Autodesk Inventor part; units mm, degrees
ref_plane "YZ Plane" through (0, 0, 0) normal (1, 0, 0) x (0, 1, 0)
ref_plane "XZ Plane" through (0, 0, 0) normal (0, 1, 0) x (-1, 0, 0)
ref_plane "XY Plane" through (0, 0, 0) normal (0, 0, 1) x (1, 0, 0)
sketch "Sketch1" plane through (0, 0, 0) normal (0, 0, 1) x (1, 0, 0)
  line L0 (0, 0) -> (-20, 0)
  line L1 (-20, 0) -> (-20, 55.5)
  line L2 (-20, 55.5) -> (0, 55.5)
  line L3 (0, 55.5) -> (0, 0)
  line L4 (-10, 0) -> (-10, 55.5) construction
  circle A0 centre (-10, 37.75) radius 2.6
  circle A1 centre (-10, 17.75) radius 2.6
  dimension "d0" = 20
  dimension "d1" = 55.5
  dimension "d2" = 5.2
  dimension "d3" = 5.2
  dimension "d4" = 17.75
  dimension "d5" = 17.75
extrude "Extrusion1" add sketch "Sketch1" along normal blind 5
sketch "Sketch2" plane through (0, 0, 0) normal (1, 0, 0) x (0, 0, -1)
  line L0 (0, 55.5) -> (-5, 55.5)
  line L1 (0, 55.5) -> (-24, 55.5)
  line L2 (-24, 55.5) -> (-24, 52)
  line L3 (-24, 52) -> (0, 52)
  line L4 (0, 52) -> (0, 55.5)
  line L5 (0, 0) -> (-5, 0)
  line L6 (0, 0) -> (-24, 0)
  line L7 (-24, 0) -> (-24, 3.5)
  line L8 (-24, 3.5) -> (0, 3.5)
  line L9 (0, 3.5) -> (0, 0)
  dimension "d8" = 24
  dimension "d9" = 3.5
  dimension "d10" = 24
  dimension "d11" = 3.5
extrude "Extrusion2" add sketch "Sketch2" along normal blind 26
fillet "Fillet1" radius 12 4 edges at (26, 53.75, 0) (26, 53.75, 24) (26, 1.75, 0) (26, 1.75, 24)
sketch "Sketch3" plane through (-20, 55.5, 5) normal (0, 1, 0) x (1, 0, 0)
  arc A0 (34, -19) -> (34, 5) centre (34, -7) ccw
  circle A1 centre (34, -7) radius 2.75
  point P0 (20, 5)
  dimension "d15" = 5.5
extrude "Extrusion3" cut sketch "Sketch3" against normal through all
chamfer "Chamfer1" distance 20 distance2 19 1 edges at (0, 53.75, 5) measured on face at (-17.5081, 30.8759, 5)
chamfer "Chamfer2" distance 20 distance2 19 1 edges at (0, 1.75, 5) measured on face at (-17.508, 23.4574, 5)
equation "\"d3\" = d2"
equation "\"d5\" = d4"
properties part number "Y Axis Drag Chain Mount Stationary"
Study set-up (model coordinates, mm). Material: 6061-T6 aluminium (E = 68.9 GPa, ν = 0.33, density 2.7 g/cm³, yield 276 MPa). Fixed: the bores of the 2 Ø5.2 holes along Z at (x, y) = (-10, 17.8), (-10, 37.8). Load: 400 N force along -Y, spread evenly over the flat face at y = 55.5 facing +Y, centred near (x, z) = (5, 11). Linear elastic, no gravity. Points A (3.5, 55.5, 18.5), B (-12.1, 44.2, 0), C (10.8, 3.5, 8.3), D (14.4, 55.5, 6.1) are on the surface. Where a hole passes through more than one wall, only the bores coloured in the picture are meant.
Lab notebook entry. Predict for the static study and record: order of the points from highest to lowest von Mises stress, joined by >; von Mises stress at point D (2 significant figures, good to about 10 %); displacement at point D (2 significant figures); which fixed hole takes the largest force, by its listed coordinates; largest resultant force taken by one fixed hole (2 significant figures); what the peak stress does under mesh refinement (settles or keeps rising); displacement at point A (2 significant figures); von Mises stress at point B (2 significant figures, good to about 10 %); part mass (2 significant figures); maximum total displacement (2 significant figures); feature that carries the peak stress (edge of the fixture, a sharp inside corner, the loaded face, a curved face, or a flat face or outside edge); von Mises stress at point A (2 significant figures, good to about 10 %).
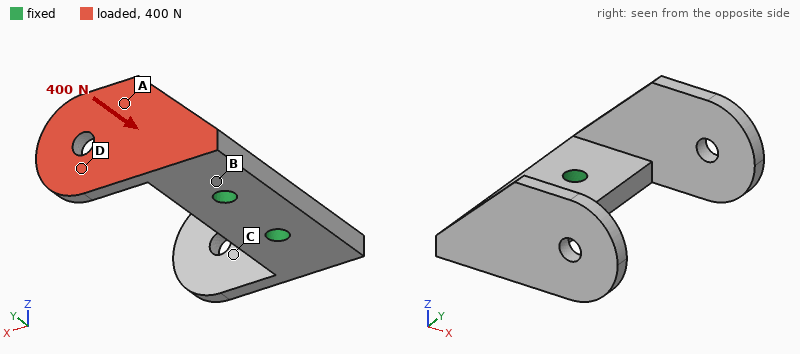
B > A > D > C
17 MPa
0.15 mm
(-10, 37.8)
390 N
keeps rising
0.16 mm
39 MPa
28 g
0.35 mm
a sharp inside corner
28 MPa
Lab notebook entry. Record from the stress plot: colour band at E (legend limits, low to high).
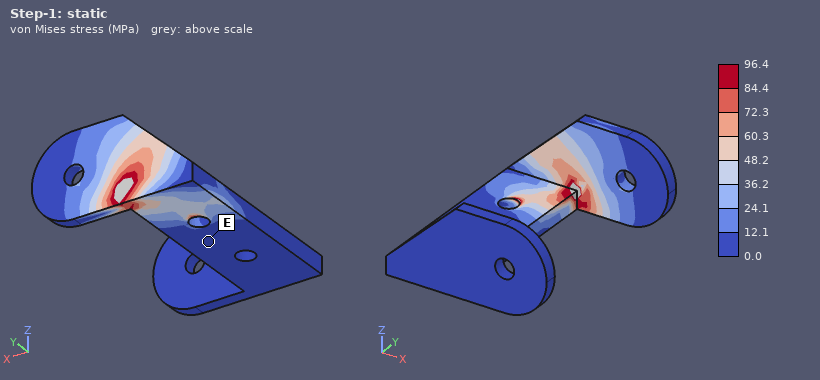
0.0 to 12.1 MPa
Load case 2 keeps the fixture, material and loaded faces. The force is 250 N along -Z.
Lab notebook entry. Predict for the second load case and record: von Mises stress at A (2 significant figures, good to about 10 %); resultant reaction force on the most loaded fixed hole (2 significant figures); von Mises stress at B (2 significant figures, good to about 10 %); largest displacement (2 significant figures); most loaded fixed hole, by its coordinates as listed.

6.0 MPa
290 N
46 MPa
0.16 mm
(-10, 37.8)
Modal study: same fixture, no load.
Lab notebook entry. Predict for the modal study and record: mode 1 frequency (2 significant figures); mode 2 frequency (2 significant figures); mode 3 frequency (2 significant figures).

2400 Hz
2400 Hz
3100 Hz
